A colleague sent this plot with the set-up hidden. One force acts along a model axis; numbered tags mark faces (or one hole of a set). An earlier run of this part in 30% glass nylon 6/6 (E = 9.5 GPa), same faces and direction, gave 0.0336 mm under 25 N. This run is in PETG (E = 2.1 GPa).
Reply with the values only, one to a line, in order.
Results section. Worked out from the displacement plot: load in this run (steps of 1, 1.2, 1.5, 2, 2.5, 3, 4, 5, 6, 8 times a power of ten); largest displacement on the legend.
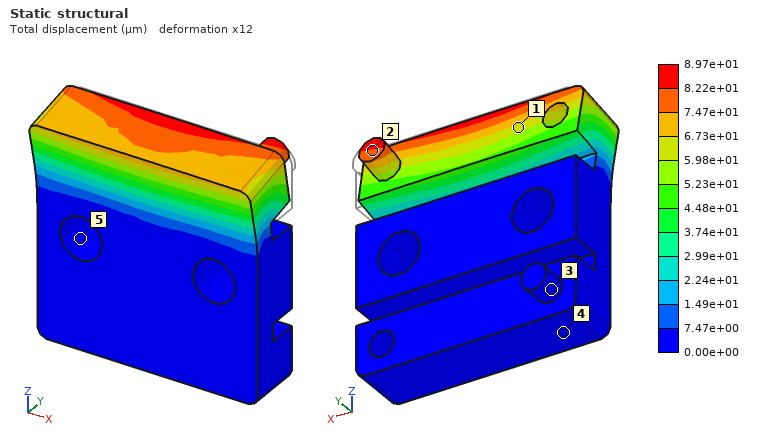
15 N
8.97e+01 µm
